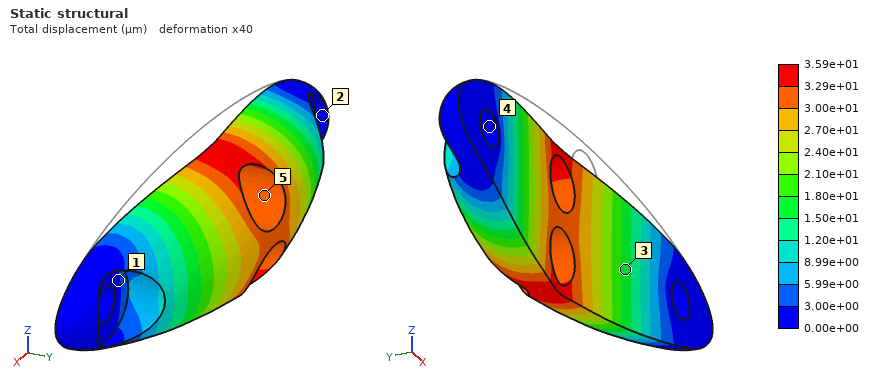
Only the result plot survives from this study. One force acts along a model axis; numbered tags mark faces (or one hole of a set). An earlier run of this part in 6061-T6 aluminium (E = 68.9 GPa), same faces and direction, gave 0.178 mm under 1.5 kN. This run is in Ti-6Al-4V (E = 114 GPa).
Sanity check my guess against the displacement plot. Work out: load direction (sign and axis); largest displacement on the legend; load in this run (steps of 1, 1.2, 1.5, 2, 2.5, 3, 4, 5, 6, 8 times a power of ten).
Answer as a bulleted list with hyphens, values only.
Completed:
- +Y
- 3.59e+01 µm
- 500 N
